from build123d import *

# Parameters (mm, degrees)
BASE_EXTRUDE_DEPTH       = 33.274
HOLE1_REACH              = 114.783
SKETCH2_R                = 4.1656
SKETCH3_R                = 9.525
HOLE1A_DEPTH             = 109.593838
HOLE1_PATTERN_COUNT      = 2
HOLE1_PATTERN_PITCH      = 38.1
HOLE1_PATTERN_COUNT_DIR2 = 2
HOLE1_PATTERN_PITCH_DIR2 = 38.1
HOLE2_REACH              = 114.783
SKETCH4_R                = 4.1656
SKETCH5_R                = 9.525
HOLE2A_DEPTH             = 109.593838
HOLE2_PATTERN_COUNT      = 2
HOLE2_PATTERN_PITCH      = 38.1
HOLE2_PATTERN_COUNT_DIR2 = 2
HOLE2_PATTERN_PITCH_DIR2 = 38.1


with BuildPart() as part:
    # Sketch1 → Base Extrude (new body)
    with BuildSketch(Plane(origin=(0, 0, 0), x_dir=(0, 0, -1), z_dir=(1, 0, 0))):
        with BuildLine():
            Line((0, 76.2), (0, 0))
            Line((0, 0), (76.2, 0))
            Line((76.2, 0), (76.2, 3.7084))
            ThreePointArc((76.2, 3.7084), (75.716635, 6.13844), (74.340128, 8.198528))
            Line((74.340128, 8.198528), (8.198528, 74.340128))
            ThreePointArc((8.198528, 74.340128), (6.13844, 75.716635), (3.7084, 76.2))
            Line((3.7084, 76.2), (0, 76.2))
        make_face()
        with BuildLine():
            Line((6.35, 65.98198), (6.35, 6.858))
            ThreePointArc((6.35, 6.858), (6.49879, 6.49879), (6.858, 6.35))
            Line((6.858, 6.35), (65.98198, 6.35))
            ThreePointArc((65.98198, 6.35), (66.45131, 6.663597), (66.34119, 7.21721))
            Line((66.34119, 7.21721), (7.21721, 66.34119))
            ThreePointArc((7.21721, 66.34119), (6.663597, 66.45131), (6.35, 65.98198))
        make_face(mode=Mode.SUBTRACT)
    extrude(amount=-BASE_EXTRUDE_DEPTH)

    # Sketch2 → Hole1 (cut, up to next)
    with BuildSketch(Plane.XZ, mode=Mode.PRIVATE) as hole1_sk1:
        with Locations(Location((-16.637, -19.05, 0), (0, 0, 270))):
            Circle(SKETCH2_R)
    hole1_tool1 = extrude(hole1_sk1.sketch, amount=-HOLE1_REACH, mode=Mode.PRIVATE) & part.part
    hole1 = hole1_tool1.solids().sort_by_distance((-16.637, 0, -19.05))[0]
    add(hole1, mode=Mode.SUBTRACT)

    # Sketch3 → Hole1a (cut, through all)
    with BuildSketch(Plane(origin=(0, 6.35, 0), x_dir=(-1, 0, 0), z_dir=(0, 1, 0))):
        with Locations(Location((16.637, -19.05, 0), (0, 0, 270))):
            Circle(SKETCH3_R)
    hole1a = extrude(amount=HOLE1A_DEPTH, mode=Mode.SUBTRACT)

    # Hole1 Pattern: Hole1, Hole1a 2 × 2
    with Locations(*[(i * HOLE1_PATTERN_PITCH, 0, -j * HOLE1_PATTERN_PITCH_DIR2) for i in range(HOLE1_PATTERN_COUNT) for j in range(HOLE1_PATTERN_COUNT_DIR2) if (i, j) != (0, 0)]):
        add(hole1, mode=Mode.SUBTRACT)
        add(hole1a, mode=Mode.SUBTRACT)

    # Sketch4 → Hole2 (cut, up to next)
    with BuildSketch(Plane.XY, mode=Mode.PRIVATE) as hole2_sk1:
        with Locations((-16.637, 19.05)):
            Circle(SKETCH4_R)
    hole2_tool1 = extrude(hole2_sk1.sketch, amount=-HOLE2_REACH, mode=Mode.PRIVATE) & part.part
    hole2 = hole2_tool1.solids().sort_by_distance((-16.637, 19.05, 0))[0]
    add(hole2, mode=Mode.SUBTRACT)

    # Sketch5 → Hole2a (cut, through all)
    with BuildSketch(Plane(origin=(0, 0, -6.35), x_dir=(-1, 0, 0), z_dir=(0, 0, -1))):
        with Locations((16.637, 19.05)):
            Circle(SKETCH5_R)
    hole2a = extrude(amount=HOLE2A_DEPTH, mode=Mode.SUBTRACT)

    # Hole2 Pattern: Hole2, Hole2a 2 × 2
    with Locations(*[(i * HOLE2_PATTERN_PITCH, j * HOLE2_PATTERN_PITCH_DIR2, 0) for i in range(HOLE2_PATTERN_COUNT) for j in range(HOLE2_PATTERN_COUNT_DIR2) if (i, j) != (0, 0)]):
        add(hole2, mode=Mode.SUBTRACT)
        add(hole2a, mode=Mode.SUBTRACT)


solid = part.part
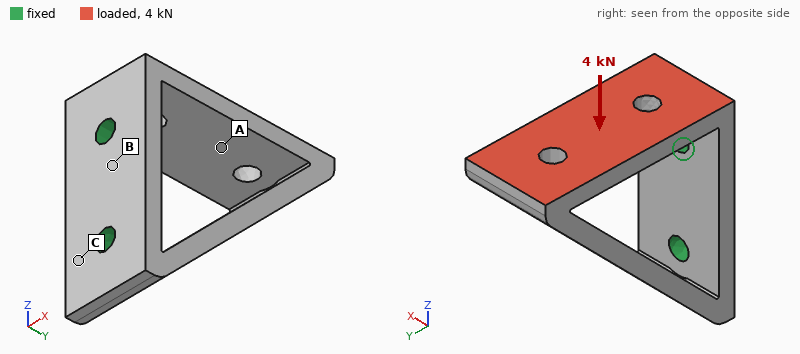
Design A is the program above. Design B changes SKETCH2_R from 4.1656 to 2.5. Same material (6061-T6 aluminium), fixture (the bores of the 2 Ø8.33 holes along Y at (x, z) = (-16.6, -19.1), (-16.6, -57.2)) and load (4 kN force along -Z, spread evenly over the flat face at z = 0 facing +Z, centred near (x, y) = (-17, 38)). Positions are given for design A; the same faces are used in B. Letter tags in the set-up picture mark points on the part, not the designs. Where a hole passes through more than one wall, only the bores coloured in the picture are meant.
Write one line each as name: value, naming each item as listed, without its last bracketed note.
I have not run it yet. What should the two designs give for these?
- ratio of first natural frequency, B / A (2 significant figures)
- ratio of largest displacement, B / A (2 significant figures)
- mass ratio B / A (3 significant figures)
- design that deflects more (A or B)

ratio of first natural frequency, B / A: 0.88
ratio of largest displacement, B / A: 1.1
mass ratio B / A: 1.01
design that deflects more: B
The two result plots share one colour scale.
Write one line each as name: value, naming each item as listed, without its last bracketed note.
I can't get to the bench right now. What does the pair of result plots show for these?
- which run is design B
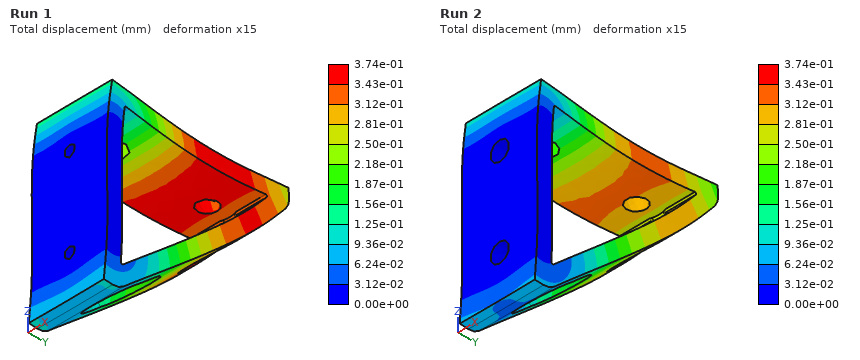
which run is design B: Run 1
